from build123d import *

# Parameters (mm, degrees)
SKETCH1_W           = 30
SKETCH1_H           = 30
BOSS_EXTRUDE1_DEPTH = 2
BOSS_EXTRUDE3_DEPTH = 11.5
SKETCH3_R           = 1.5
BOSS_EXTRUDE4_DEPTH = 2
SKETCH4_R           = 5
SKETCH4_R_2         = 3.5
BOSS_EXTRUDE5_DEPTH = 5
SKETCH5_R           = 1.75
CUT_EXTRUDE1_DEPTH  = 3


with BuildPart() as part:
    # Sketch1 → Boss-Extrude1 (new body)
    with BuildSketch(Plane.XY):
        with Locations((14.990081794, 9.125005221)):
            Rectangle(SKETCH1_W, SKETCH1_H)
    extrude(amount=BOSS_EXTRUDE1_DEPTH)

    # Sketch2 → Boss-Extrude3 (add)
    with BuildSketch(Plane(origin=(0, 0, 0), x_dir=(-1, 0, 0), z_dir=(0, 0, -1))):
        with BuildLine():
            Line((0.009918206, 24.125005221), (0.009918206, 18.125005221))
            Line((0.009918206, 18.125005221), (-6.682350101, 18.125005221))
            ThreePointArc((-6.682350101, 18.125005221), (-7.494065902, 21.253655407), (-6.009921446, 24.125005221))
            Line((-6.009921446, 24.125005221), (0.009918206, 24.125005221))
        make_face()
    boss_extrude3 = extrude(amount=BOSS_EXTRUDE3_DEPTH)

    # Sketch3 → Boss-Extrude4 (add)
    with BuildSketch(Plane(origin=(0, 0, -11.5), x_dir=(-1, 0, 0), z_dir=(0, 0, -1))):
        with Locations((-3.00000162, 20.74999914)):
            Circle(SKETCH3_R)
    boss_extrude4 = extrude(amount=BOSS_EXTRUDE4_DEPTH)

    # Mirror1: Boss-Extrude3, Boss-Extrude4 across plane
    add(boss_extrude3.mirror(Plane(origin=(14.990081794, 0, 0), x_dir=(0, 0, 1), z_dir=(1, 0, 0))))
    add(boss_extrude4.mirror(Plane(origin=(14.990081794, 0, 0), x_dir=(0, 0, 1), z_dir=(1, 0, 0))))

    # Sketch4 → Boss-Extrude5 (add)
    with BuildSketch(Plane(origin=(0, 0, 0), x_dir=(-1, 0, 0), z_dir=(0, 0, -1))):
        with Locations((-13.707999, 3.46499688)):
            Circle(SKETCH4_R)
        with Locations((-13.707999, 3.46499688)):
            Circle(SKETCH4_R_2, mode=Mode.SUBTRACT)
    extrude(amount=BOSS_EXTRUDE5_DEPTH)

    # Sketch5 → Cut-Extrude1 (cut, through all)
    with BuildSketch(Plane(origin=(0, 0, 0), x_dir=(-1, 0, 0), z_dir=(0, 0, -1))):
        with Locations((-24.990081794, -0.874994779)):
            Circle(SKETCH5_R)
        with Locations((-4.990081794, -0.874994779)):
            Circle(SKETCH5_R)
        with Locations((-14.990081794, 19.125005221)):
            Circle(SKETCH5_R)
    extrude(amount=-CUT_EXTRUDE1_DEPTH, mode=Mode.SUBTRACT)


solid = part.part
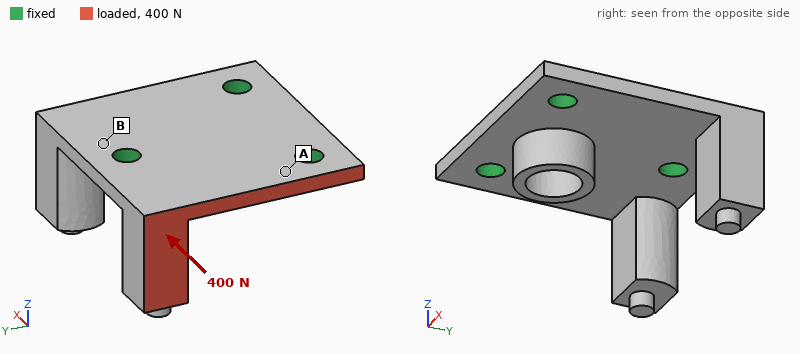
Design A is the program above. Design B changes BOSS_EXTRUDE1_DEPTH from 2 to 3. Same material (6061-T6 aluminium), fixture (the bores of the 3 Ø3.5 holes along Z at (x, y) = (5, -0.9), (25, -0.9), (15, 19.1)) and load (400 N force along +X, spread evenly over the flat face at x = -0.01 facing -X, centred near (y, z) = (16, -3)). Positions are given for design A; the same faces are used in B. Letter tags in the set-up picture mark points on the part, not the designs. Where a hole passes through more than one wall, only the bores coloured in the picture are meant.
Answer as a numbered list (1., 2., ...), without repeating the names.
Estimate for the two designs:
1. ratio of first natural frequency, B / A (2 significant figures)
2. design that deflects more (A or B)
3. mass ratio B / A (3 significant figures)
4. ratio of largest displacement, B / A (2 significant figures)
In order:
1. 1.6
2. A
3. 1.29
4. 0.31
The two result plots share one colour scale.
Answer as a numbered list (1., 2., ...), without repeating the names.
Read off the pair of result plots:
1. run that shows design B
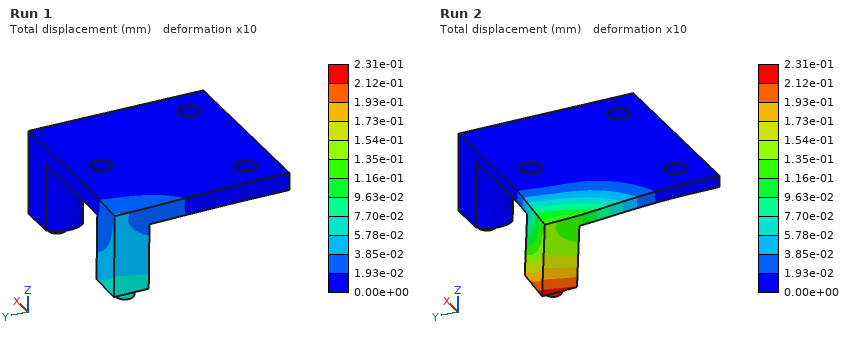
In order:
1. Run 1
